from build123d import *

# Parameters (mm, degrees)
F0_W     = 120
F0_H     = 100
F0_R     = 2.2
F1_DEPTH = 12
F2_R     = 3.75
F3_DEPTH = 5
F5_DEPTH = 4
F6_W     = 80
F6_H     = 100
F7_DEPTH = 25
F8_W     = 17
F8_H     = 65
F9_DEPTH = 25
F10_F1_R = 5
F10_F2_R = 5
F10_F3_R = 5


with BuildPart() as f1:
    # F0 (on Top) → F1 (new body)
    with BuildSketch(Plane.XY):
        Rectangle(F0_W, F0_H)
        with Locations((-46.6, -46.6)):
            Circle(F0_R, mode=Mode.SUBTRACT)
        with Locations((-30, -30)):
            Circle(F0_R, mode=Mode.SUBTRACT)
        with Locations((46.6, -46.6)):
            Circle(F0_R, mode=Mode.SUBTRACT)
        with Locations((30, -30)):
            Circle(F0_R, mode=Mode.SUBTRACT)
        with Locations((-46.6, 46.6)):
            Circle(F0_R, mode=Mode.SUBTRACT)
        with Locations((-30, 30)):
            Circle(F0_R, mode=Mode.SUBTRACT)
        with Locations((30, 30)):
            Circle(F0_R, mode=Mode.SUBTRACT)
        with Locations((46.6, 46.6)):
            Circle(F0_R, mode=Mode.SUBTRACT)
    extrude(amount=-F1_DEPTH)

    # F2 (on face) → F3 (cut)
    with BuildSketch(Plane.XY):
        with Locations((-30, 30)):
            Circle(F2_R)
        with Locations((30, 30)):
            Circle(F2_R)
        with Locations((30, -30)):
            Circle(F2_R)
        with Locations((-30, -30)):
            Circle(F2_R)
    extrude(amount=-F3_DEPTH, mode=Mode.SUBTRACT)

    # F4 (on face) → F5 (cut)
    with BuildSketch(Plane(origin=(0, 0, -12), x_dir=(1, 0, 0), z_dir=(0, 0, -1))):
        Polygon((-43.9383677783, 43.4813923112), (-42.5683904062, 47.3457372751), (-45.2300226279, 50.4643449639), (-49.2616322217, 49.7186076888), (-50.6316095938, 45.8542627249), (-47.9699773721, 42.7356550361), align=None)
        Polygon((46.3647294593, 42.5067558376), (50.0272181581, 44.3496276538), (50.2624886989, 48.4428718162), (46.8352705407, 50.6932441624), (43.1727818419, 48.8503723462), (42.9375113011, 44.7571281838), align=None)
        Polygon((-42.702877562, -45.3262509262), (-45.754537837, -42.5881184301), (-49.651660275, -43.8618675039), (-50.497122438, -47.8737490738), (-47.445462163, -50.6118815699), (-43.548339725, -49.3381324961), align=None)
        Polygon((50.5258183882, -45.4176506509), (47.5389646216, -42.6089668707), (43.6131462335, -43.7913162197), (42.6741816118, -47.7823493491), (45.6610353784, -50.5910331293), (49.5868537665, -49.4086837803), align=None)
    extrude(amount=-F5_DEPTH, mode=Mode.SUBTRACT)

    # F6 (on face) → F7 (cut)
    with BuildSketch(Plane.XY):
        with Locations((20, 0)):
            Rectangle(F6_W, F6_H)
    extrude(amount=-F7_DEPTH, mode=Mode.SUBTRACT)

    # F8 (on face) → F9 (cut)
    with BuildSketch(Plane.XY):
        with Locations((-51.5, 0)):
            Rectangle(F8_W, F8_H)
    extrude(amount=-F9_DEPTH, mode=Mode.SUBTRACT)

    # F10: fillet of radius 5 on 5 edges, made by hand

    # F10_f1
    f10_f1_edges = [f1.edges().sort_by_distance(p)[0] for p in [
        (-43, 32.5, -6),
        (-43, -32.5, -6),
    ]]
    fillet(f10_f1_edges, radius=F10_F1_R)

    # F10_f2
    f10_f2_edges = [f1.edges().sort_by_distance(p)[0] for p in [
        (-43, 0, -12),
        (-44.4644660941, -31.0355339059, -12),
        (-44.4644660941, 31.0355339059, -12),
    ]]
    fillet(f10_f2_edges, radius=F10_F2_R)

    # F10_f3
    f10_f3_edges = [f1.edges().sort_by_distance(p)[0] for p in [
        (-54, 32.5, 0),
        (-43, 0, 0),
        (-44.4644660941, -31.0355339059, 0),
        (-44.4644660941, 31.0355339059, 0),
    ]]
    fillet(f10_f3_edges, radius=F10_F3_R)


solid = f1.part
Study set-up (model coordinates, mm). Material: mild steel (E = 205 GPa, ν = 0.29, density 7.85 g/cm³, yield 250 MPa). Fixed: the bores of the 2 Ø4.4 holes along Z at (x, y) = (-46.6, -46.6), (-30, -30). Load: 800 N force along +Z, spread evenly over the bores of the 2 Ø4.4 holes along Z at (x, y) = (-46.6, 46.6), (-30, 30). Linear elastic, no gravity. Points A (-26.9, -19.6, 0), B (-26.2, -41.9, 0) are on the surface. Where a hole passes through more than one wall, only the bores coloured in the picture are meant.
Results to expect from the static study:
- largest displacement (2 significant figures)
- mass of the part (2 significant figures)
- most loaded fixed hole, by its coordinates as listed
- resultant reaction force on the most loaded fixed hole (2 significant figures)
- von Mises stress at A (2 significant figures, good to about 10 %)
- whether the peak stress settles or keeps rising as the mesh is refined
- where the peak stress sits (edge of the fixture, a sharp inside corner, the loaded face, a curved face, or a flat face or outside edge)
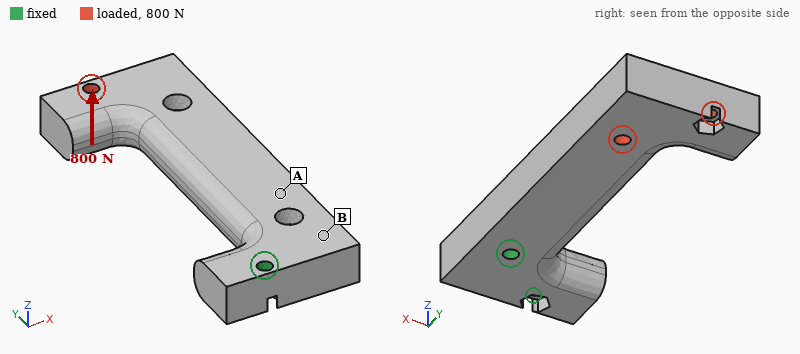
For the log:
0.26 mm
260 g
(-30, -30)
1.9 kN
85 MPa
keeps rising
edge of the fixture
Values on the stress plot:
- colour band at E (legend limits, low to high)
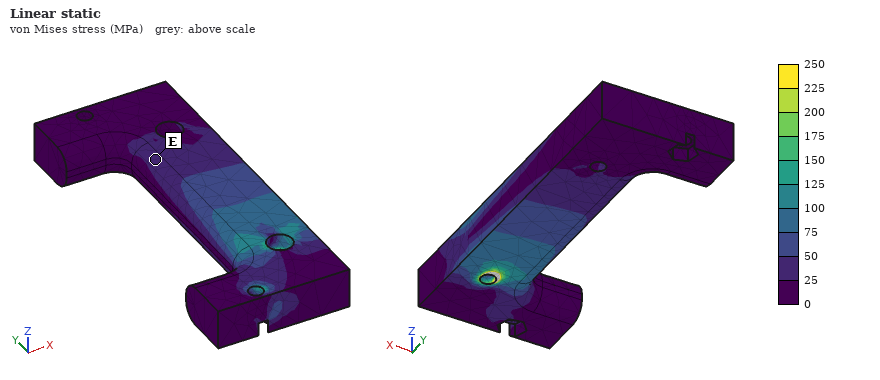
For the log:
25 to 50 MPa
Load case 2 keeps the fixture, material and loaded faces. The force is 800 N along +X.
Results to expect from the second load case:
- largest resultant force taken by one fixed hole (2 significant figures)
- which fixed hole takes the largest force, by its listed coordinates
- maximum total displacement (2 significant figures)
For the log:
2.5 kN
(-30, -30)
82 µm
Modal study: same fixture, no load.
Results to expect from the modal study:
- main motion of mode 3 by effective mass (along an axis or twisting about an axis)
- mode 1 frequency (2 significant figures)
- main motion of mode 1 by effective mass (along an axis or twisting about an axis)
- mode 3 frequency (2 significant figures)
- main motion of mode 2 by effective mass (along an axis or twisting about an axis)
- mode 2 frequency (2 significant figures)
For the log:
twisting about Y
1000 Hz
along Z
4200 Hz
along X
1800 Hz
